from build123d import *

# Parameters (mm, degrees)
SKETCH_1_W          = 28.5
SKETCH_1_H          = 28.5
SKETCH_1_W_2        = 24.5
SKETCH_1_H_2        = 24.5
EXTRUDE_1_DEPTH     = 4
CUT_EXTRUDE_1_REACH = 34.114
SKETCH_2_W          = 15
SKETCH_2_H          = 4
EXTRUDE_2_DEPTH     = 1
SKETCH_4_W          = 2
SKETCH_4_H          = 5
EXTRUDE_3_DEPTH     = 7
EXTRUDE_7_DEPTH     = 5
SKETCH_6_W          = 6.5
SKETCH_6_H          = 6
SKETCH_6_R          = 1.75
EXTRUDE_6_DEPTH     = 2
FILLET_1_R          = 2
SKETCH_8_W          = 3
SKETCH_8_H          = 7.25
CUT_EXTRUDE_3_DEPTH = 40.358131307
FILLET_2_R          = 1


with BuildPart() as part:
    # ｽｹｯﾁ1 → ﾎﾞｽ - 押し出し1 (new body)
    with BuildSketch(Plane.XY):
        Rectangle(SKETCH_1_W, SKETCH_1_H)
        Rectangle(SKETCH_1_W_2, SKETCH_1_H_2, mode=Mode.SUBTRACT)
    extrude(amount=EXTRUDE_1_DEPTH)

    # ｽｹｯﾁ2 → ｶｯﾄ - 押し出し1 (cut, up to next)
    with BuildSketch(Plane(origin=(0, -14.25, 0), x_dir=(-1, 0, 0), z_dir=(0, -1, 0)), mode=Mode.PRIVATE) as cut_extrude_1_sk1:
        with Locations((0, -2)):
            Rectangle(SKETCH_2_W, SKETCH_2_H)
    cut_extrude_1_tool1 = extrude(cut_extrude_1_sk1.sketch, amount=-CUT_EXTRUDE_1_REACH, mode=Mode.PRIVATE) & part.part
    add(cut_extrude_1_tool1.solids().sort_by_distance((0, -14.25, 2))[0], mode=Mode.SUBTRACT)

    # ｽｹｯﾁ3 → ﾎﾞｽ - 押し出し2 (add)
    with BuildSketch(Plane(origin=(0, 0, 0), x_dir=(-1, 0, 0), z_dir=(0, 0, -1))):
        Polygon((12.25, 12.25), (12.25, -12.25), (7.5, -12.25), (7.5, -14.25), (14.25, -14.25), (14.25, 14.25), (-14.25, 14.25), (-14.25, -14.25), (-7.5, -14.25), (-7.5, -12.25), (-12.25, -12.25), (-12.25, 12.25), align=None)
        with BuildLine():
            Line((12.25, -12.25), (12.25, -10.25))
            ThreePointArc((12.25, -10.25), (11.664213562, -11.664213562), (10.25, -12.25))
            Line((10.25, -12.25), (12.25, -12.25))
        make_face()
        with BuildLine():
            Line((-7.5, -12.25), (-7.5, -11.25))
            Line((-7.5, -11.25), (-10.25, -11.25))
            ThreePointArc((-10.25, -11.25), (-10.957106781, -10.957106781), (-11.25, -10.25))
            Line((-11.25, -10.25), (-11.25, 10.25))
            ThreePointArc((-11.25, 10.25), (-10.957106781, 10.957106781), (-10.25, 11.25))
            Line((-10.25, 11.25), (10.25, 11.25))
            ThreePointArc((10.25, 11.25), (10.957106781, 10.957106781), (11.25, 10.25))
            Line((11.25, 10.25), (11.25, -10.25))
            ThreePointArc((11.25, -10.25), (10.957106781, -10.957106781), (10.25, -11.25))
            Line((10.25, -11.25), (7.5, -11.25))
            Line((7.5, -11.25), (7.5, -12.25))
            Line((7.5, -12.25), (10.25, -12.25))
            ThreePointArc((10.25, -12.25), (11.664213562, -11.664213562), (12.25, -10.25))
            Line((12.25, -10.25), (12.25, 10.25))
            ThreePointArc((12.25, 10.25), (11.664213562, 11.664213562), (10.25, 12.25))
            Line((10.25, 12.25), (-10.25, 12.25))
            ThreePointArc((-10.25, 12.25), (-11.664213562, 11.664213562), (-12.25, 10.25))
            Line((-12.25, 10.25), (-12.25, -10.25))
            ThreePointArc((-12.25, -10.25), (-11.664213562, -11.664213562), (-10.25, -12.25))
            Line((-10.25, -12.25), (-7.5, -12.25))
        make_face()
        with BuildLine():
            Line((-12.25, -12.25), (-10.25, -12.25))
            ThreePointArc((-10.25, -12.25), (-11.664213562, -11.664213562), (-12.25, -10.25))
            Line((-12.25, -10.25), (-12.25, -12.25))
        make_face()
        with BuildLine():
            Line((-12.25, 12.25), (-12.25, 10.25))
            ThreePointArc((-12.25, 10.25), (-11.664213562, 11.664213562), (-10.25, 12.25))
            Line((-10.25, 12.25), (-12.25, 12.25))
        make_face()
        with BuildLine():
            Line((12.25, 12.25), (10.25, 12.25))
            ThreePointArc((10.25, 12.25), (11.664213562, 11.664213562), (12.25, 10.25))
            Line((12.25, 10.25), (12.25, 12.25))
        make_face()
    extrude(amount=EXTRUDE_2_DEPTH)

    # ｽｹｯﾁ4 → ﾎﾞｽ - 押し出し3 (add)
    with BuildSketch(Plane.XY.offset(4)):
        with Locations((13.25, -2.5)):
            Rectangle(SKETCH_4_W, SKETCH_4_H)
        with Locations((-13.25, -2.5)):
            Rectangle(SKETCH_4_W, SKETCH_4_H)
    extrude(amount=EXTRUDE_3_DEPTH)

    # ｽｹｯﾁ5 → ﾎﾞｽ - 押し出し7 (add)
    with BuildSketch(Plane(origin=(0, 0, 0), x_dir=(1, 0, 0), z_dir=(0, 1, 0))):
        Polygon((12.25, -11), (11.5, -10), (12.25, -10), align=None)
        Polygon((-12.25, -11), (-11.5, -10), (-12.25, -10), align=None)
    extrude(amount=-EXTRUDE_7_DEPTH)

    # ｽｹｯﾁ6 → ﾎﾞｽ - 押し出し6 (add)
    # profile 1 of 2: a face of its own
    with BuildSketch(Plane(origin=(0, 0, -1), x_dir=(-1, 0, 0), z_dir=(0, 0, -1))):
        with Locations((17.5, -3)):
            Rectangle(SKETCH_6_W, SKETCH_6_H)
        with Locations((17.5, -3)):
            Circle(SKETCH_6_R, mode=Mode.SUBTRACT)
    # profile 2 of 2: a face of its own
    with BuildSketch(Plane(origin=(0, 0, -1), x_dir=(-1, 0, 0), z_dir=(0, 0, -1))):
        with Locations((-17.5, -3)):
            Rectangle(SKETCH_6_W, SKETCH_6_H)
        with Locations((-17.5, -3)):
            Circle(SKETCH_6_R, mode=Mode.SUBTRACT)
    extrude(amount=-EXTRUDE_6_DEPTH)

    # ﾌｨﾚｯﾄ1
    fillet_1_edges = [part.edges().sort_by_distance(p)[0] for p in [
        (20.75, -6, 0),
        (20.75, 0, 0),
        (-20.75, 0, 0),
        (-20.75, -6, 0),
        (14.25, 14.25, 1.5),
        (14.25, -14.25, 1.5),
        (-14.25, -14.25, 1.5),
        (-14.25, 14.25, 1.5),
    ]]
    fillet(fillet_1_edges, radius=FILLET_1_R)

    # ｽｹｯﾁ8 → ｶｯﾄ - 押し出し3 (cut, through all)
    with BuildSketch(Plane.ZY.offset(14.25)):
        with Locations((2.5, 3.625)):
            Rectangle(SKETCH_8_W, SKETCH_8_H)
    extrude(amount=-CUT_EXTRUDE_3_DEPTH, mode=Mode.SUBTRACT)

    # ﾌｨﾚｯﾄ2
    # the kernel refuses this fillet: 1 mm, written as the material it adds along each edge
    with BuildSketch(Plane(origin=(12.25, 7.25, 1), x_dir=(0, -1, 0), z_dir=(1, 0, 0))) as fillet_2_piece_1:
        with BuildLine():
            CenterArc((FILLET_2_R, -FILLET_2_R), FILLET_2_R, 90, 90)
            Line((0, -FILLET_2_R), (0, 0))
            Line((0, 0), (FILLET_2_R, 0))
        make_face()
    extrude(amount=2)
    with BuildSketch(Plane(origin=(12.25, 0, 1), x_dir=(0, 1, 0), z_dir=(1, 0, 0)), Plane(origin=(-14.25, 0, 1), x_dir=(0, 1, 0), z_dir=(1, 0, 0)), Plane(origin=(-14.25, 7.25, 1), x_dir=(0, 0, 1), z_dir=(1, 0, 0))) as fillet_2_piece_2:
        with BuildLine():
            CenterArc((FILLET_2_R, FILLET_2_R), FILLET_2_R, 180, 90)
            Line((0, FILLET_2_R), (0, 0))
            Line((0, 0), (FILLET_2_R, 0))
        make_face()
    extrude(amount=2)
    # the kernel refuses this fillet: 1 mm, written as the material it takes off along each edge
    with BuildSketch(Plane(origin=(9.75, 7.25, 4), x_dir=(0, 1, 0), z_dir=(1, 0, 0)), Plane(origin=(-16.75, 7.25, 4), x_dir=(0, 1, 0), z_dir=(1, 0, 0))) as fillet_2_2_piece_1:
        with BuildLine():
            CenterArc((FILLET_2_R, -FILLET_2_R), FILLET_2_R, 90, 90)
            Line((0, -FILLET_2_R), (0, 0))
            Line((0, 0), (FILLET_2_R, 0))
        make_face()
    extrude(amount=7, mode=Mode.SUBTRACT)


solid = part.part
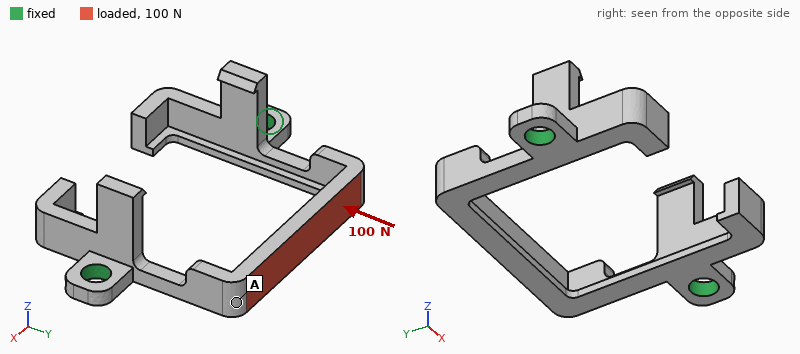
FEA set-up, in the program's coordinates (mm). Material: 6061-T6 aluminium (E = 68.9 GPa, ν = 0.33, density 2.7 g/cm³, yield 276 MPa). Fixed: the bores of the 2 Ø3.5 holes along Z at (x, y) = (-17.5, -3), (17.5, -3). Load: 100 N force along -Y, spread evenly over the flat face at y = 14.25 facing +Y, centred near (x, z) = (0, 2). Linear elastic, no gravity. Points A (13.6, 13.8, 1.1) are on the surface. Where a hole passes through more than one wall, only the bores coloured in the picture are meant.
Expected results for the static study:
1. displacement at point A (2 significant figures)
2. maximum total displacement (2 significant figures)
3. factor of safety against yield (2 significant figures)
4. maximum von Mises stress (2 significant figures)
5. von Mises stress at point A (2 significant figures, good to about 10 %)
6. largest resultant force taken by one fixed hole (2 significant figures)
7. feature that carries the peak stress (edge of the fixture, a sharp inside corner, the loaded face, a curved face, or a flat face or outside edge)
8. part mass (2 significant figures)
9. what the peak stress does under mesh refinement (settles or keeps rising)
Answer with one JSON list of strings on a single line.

["68 µm", "96 µm", "2.4", "120 MPa", "12 MPa", "54 N", "a curved face", "3.1 g", "settles"]
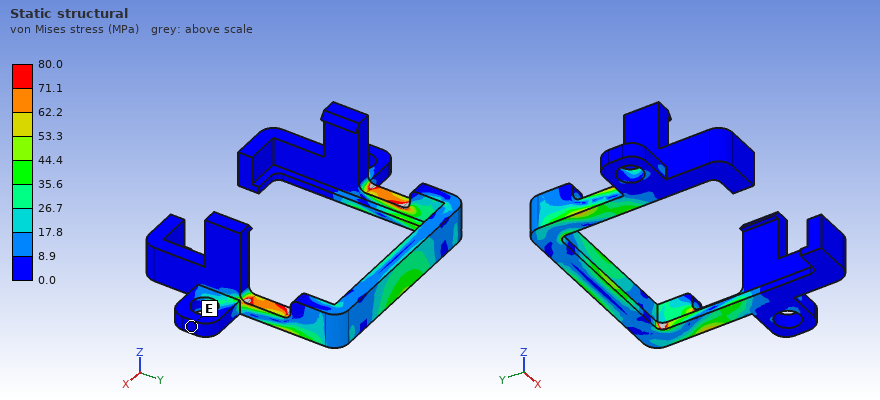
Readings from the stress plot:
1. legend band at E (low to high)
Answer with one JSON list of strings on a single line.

["0.0 to 8.9 MPa"]
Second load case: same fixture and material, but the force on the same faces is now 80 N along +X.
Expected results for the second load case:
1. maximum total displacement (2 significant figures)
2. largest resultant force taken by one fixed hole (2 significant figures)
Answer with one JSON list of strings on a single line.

["70 µm", "48 N"]
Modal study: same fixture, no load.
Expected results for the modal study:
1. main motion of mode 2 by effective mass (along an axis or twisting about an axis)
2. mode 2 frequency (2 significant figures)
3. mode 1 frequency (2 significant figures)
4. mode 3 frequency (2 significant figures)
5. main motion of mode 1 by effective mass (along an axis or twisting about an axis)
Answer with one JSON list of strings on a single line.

["along X", "5100 Hz", "2400 Hz", "6200 Hz", "along Z"]
